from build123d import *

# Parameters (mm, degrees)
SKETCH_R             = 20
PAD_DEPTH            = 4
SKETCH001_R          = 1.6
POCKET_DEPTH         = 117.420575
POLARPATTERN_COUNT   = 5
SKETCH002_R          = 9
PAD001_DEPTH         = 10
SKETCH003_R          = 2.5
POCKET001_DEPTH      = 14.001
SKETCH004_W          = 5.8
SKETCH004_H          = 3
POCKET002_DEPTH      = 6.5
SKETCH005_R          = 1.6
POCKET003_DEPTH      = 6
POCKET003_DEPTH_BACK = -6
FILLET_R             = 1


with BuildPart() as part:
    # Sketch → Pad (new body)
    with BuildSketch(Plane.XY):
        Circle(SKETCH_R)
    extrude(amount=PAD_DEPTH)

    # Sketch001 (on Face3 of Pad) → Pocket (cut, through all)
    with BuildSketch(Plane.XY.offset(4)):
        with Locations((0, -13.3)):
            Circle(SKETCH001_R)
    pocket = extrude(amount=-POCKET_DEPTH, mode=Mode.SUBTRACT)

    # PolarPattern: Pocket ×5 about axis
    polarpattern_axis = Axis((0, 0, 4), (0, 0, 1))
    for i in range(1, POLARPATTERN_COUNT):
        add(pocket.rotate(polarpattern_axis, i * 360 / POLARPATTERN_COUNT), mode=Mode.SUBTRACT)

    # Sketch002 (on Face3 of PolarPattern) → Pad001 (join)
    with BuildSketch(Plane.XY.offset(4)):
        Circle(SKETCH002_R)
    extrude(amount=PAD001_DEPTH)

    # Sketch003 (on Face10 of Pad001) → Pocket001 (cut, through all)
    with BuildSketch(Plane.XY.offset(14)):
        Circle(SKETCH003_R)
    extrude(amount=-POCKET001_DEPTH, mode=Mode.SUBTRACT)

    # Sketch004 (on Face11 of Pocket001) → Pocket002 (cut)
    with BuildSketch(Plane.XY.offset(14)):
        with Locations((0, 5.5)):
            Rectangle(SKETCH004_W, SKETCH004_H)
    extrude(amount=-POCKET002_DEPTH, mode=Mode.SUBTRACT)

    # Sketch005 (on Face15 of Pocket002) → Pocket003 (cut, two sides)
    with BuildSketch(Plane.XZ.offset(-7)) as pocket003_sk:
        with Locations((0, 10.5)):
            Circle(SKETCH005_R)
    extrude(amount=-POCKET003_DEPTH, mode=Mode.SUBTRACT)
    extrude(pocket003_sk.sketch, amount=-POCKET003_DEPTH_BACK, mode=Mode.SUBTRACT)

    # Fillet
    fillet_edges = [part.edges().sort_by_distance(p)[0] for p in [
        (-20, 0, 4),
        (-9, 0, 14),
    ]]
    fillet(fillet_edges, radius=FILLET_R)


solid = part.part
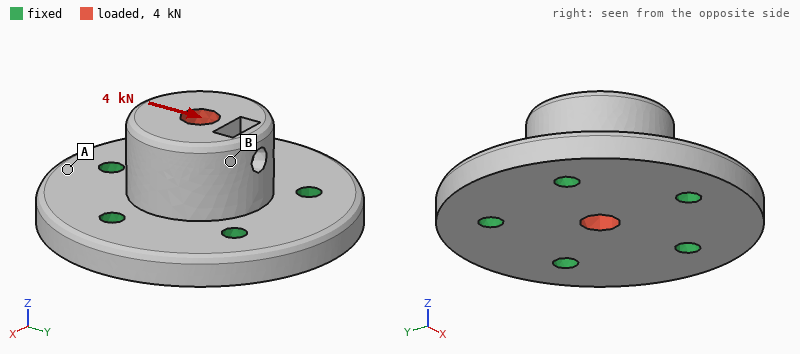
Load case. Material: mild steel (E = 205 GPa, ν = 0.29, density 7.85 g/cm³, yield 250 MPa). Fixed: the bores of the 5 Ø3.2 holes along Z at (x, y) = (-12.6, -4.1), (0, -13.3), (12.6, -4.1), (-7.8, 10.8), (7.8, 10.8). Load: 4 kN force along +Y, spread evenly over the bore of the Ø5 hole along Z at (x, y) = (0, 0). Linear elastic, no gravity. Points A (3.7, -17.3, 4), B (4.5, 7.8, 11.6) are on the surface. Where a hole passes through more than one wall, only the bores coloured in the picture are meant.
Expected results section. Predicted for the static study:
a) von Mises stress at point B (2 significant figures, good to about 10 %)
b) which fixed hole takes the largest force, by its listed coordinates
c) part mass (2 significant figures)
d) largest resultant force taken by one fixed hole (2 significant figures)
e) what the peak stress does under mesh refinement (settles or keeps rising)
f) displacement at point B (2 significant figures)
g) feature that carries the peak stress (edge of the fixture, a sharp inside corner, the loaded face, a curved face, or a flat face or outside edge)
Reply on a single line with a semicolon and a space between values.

17 MPa; (0, -13.3); 55 g; 1.3 kN; keeps rising; 3.8 µm; edge of the fixture
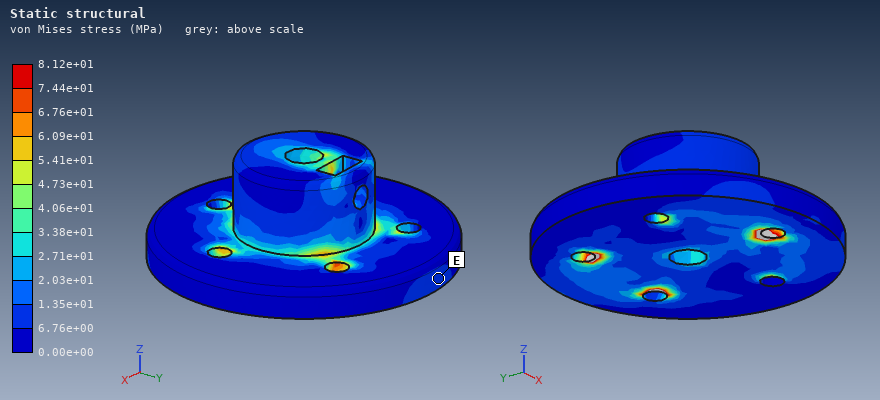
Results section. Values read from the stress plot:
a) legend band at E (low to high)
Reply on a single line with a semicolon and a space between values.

6.76e+00 to 1.35e+01 MPa
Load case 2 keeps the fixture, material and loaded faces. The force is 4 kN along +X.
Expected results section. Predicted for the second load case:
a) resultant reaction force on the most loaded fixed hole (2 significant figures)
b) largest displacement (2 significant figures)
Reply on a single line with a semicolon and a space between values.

1.3 kN; 4.8 µm
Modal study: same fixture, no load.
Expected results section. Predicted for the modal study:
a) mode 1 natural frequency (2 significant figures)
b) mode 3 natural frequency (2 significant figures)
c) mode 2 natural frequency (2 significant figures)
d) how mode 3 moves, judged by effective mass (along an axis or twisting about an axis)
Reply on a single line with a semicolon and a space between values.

34 kHz; 37 kHz; 34 kHz; along Z
